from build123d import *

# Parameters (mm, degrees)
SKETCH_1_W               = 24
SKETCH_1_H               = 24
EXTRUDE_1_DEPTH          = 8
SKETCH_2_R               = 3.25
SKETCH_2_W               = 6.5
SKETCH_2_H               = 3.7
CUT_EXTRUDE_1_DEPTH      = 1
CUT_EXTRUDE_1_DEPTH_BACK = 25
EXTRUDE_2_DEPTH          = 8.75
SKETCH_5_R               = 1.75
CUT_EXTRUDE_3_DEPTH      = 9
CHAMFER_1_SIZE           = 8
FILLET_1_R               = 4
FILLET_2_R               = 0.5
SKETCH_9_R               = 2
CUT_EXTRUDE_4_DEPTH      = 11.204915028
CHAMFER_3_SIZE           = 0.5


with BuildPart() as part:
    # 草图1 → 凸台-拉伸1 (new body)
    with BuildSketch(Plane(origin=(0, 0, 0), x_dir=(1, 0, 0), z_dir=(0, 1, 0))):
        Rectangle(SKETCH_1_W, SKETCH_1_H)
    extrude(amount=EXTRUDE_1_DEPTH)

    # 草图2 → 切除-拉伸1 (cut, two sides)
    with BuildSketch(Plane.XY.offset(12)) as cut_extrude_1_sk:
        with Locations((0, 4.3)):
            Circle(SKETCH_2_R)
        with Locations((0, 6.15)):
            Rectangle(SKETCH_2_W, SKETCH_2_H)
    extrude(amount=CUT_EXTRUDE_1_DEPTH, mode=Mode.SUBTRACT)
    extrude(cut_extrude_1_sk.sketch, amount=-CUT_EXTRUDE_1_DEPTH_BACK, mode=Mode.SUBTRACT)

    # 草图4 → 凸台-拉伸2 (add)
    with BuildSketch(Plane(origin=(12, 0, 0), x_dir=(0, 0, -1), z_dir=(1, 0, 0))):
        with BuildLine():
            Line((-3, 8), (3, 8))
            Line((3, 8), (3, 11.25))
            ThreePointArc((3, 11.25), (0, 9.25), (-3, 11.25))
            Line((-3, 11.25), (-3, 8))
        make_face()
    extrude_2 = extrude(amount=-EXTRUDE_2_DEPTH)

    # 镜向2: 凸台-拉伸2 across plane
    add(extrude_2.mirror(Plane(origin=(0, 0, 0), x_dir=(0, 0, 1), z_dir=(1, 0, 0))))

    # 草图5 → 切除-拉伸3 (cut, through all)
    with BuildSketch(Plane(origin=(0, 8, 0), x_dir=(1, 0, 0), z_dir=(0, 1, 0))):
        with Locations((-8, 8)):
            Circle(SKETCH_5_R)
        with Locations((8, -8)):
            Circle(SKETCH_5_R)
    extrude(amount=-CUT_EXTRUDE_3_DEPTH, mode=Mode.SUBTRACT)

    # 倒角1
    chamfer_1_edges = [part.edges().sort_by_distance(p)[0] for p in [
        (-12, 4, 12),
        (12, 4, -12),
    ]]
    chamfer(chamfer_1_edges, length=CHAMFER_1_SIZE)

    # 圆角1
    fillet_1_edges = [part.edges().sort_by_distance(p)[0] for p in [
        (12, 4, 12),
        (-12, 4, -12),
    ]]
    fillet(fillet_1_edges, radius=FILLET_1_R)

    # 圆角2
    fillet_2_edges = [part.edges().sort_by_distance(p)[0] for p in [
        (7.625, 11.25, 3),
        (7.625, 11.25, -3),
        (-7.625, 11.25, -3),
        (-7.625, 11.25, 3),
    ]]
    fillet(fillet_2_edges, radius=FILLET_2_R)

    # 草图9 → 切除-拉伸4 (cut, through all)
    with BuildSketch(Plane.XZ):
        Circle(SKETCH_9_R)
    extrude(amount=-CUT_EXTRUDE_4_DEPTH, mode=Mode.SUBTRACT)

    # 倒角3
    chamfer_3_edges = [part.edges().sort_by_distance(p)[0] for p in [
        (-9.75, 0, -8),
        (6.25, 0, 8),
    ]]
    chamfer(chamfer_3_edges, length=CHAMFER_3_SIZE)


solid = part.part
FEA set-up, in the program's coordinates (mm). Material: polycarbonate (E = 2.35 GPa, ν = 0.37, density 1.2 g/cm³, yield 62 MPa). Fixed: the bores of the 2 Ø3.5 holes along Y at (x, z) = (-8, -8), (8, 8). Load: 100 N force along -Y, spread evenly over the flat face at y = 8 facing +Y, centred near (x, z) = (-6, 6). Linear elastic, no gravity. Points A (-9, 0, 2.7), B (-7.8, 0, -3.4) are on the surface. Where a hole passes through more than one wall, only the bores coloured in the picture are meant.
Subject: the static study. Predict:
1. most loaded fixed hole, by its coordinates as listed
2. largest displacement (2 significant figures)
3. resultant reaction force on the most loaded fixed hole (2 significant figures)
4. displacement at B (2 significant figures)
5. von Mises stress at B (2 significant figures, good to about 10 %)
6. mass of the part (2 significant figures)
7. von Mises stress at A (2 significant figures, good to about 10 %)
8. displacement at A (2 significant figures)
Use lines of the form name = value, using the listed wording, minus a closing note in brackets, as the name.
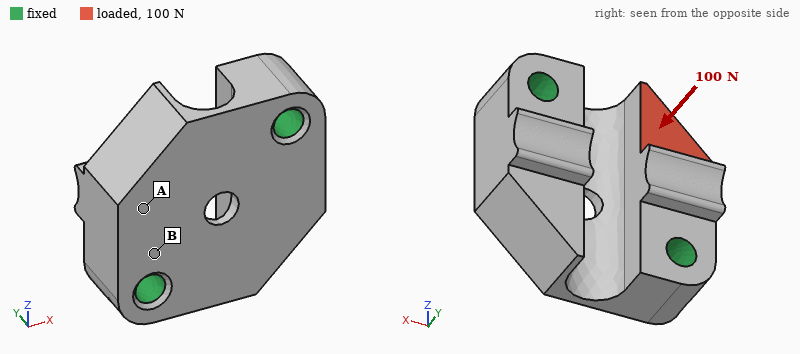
most loaded fixed hole, by its coordinates as listed = (-8, -8)
largest displacement = 0.13 mm
resultant reaction force on the most loaded fixed hole = 82 N
displacement at B = 0.022 mm
von Mises stress at B = 6.5 MPa
mass of the part = 3.7 g
von Mises stress at A = 2.3 MPa
displacement at A = 0.063 mm
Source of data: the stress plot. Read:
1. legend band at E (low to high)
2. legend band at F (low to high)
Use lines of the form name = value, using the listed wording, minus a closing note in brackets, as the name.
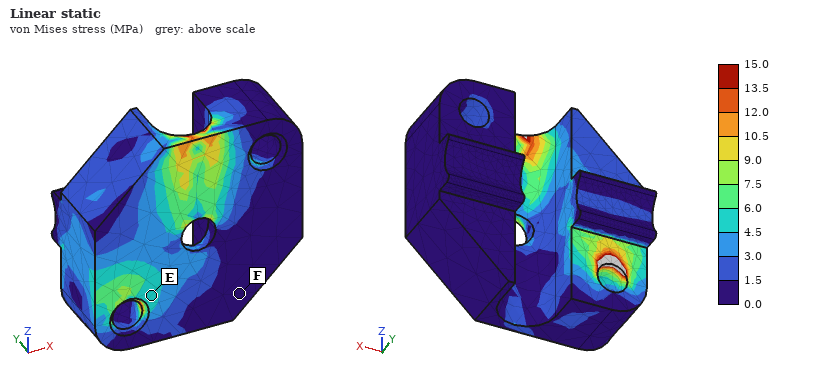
legend band at E = 4.5 to 6.0 MPa
legend band at F = 0.0 to 1.5 MPa
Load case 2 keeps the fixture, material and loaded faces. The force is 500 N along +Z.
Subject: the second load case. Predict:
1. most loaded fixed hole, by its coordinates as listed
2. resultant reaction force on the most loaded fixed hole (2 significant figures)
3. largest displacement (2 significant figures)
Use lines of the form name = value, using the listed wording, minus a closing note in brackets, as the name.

most loaded fixed hole, by its coordinates as listed = (-8, -8)
resultant reaction force on the most loaded fixed hole = 500 N
largest displacement = 0.39 mm
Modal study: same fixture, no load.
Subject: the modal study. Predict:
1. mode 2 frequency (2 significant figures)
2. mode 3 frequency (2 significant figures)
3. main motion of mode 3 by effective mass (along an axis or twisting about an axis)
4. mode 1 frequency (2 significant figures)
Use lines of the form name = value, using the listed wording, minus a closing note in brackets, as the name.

mode 2 frequency = 6700 Hz
mode 3 frequency = 8800 Hz
main motion of mode 3 by effective mass = along X
mode 1 frequency = 6400 Hz
